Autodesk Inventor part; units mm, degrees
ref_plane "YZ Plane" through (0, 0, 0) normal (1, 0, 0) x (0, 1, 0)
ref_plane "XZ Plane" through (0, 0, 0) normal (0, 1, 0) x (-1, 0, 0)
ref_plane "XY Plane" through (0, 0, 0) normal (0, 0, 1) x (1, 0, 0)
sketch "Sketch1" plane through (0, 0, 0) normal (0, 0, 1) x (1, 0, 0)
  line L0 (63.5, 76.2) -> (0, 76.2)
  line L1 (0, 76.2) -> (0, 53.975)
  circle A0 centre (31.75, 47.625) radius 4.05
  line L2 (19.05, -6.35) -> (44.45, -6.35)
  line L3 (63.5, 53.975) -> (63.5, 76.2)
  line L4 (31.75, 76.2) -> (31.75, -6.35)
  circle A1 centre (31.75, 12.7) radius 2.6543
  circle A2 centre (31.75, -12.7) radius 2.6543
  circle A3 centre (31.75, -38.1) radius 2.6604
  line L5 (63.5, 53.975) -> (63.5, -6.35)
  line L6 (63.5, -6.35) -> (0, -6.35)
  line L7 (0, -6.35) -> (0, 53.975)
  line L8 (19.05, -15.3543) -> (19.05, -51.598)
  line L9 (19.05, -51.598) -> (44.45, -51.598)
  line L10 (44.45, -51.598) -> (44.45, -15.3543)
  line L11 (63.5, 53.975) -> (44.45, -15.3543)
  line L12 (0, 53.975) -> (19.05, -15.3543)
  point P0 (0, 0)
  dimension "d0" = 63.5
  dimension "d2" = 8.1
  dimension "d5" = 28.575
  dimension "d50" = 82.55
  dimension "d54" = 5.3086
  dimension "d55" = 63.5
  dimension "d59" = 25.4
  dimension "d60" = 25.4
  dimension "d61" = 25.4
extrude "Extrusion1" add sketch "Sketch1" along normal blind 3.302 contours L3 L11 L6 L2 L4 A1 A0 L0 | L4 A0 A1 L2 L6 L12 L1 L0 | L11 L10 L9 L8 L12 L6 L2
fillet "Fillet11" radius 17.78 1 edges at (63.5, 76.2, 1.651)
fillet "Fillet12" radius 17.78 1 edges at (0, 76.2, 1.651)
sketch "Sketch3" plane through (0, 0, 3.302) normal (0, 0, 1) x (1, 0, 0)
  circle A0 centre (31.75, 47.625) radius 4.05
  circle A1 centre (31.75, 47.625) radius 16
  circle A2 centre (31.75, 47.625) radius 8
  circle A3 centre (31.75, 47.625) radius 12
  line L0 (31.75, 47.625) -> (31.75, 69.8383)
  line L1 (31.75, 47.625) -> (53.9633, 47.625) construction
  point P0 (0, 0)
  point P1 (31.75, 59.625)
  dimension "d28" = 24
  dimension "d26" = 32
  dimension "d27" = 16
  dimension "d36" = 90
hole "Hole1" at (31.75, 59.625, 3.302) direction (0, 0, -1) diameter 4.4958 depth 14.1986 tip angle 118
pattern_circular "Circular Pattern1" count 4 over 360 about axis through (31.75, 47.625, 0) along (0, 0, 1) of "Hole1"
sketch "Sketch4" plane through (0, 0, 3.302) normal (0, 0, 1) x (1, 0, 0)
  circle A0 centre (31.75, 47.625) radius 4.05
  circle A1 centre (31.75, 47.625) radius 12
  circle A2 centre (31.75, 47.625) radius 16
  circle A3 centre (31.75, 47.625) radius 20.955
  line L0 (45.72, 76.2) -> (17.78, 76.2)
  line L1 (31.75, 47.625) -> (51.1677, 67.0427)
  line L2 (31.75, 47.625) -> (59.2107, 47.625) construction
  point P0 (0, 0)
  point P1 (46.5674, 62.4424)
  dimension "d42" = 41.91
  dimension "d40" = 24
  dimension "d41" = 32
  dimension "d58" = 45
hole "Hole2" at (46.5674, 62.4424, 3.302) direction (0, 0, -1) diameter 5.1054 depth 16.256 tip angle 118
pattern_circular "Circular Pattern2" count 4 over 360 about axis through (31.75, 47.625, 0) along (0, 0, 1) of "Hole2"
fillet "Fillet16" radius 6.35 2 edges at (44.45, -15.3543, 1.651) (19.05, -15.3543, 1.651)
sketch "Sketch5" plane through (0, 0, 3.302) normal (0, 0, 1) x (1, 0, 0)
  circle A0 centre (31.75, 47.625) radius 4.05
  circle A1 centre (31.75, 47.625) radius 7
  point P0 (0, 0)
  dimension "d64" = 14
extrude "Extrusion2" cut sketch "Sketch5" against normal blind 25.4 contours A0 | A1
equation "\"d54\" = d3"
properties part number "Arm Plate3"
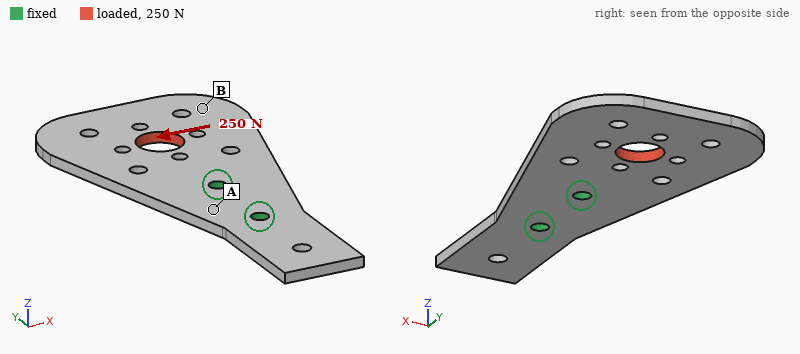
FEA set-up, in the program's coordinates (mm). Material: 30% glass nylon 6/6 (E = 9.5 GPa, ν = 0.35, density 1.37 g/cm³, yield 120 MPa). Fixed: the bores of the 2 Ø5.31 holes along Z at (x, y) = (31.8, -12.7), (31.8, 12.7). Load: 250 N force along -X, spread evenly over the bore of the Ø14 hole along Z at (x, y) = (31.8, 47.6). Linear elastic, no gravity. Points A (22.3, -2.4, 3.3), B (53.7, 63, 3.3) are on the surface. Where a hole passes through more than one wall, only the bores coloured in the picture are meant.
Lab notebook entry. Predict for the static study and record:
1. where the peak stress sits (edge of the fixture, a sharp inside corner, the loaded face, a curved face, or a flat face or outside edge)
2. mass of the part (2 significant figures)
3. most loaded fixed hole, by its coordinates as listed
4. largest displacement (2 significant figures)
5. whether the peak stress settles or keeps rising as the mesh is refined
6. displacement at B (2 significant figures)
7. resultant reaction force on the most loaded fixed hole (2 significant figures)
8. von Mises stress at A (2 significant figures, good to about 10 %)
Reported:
edge of the fixture
22 g
(31.8, 12.7)
0.16 mm
keeps rising
0.14 mm
520 N
5.5 MPa
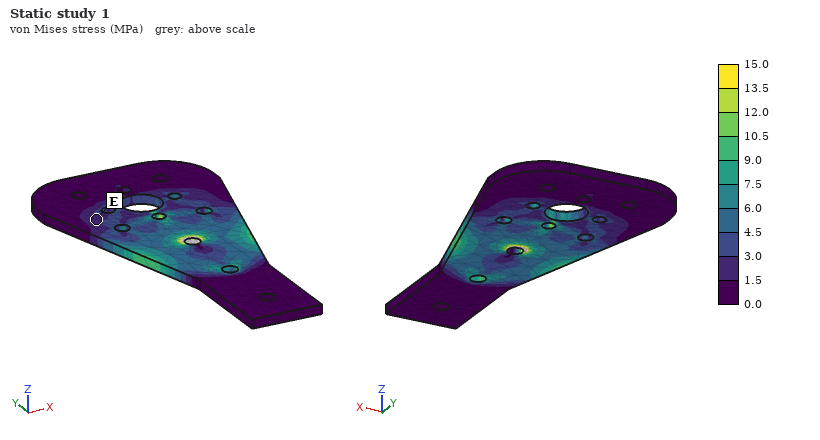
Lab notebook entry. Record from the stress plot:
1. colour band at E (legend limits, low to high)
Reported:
1.5 to 3.0 MPa
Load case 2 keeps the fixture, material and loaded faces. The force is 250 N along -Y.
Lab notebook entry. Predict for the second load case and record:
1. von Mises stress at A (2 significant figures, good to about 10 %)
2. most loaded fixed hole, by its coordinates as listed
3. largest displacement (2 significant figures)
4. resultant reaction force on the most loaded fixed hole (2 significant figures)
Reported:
0.94 MPa
(31.8, 12.7)
15 µm
190 N
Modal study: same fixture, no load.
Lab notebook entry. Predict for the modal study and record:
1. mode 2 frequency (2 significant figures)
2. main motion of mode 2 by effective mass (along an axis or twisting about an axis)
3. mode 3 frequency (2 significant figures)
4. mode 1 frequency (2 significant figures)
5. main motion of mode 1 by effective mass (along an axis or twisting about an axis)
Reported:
620 Hz
twisting about Y
990 Hz
310 Hz
along Z
